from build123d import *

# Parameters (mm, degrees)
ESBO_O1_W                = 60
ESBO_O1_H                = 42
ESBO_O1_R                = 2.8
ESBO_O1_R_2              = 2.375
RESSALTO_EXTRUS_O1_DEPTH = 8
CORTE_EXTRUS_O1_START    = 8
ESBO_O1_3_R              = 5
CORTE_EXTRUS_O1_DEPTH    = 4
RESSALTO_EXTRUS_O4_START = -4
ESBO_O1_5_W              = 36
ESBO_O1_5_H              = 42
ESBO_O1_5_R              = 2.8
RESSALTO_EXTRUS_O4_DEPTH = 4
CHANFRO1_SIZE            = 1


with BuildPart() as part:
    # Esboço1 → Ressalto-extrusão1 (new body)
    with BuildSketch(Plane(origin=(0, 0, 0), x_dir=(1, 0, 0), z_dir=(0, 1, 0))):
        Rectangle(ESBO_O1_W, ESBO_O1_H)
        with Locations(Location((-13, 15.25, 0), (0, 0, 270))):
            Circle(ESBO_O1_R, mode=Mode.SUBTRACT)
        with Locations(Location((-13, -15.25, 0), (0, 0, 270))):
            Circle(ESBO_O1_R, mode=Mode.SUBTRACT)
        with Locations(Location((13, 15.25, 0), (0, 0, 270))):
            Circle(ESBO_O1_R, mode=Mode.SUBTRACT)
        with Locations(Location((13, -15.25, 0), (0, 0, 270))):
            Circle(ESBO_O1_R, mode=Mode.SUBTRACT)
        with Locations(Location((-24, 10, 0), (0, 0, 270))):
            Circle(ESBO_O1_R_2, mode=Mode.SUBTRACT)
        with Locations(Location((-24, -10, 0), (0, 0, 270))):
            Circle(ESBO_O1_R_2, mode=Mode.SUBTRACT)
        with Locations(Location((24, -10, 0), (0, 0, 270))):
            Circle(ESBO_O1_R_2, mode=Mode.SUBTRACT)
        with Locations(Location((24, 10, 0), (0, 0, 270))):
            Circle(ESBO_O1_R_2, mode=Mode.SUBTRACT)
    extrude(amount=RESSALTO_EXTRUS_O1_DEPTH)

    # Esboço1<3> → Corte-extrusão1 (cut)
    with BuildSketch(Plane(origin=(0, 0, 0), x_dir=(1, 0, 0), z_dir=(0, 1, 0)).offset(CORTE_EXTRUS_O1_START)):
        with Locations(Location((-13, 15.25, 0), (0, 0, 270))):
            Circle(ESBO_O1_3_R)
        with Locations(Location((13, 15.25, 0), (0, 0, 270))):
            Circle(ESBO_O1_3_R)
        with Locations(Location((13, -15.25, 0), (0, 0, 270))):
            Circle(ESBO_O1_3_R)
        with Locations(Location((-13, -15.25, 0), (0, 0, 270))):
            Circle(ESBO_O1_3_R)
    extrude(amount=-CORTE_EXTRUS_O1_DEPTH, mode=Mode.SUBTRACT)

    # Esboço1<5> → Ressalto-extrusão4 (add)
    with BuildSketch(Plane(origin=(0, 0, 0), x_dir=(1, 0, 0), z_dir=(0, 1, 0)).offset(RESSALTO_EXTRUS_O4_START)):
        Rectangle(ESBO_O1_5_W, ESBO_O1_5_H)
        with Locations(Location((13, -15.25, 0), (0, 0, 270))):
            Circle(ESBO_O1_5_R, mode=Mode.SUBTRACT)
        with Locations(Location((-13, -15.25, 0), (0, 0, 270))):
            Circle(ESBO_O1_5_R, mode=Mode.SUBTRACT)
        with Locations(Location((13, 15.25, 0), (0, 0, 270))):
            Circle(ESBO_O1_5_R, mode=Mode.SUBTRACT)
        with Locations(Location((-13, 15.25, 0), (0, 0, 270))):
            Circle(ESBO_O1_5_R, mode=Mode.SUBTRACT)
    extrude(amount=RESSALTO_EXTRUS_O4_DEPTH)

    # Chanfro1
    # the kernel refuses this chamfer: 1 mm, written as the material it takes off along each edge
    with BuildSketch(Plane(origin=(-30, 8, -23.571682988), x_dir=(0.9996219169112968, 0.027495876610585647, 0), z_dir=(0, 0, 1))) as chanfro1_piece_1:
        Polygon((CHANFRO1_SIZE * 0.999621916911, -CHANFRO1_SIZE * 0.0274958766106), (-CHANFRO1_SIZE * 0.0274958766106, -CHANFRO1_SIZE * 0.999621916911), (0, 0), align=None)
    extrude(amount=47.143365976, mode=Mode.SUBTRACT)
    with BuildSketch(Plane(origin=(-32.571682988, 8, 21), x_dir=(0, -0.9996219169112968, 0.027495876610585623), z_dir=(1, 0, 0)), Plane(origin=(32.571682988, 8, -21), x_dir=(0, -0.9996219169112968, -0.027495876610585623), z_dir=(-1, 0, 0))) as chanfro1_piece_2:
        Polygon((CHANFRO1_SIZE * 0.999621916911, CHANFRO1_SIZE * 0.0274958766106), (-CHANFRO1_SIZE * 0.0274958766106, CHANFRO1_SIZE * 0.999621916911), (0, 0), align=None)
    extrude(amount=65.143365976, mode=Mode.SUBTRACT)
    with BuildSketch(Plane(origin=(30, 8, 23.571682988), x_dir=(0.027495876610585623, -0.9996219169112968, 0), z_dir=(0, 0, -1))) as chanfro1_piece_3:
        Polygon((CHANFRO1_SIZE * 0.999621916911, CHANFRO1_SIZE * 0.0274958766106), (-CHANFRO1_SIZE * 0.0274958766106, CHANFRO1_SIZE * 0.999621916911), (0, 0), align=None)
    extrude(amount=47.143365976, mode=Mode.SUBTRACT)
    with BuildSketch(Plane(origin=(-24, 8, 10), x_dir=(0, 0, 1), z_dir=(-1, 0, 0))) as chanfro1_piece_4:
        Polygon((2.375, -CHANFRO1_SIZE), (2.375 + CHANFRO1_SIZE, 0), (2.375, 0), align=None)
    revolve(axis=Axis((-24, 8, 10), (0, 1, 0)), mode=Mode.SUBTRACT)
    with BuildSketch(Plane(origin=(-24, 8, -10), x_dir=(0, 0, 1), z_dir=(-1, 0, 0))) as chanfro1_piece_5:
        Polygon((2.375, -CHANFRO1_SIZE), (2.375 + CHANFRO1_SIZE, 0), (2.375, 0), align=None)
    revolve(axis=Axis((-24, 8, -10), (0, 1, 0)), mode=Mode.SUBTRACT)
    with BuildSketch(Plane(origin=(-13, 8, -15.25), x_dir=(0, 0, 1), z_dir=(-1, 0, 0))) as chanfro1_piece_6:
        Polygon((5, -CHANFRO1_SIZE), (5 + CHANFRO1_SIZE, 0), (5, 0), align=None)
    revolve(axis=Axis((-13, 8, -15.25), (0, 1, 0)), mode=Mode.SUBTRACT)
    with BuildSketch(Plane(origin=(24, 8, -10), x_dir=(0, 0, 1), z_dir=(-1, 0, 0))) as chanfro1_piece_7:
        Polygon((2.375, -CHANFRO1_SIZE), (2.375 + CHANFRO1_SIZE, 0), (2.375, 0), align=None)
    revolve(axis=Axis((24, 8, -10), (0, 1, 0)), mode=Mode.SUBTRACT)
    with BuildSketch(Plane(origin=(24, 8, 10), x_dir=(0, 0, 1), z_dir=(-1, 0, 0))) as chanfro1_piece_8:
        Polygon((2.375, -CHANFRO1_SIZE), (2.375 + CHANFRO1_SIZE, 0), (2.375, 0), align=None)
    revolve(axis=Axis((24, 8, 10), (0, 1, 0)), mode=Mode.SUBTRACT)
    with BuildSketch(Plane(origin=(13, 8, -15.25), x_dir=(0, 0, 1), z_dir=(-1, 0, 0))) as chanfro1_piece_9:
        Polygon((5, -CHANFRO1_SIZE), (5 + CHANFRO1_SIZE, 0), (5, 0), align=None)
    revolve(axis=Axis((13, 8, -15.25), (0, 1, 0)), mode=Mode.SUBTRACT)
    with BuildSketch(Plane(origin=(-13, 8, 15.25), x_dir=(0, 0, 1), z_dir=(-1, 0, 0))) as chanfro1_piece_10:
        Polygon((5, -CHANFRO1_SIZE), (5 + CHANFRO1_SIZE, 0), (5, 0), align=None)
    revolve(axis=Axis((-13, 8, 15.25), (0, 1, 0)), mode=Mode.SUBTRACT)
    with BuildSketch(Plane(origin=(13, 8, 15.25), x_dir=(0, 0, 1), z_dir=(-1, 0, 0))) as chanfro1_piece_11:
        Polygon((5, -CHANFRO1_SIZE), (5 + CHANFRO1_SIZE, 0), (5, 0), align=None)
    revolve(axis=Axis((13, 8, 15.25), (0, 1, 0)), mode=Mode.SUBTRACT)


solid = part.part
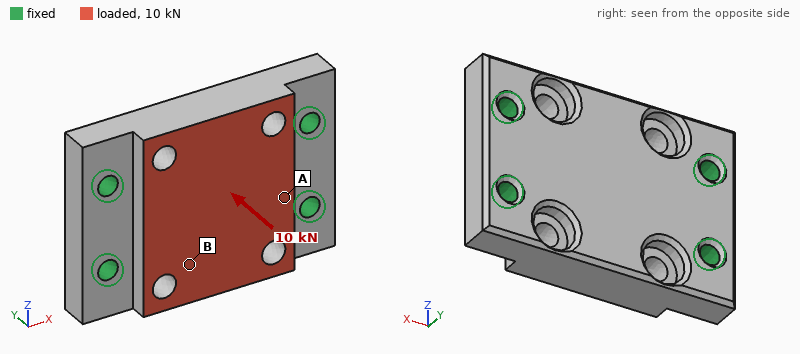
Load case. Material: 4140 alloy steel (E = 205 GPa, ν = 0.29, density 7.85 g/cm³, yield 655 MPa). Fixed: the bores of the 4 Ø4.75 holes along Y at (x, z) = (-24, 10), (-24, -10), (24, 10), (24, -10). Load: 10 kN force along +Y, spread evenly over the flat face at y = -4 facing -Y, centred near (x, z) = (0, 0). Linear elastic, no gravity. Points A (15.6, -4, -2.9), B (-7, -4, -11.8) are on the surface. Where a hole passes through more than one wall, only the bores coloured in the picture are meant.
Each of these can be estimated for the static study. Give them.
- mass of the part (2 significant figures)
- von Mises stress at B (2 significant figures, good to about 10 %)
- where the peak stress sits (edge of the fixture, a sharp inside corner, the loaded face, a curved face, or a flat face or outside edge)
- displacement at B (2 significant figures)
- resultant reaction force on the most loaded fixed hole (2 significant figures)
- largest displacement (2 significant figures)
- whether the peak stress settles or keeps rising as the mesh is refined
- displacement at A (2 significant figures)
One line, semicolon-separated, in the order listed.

180 g; 42 MPa; edge of the fixture; 9.2 µm; 2.8 kN; 12 µm; keeps rising; 5.5 µm
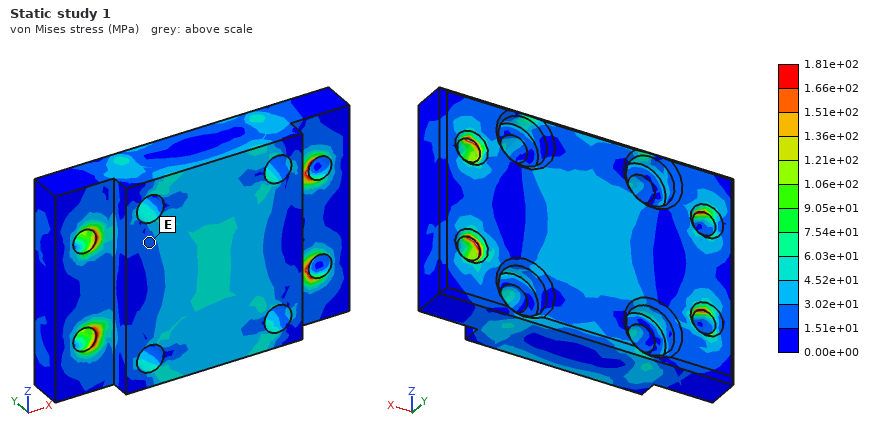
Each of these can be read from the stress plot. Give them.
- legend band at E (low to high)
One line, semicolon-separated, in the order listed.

1.51e+01 to 3.02e+01 MPa
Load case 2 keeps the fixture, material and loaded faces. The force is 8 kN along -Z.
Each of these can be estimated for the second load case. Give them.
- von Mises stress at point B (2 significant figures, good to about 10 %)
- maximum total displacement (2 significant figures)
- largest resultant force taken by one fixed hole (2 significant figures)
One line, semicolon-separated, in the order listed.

16 MPa; 9.6 µm; 2.7 kN
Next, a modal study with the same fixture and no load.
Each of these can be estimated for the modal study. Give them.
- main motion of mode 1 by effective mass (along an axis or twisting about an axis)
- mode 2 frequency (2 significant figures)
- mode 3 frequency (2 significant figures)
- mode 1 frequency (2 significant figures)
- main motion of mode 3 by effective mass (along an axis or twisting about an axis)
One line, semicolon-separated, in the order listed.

along Y; 16 kHz; 24 kHz; 15 kHz; along Z
